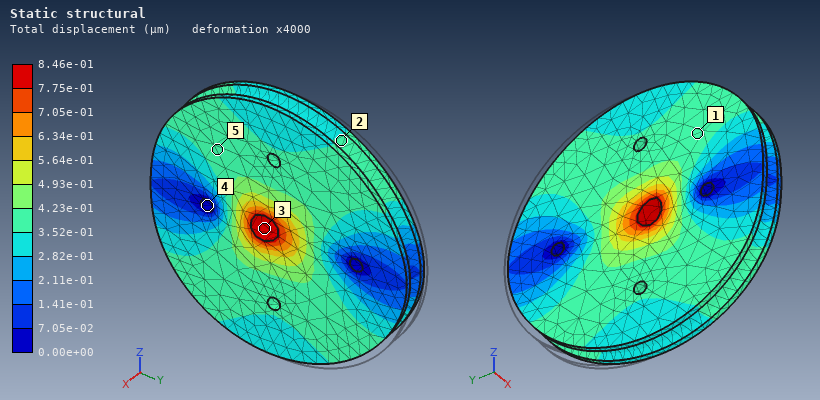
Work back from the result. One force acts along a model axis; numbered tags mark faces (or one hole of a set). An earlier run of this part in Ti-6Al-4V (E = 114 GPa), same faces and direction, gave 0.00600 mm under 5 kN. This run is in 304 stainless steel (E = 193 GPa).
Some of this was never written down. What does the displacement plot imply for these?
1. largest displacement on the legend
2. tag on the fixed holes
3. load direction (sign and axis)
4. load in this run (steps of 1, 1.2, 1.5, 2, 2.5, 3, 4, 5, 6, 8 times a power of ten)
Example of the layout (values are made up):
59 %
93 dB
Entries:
8.46e-01 µm
4
-Y
1.2 kN
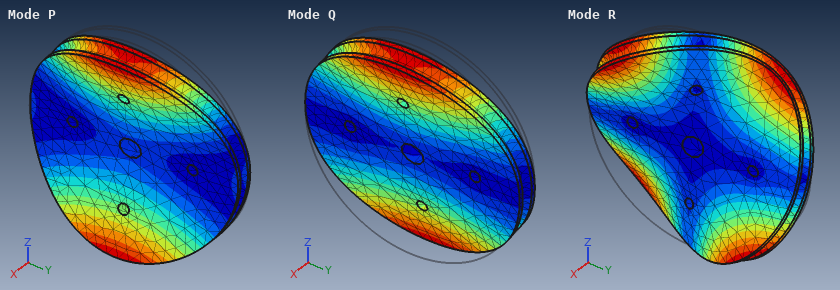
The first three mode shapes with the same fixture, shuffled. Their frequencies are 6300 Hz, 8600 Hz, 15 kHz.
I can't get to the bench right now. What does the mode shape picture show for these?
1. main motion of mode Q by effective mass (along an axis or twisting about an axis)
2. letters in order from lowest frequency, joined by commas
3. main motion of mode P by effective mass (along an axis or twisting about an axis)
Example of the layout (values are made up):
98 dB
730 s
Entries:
twisting about Y
Q, P, R
along X
